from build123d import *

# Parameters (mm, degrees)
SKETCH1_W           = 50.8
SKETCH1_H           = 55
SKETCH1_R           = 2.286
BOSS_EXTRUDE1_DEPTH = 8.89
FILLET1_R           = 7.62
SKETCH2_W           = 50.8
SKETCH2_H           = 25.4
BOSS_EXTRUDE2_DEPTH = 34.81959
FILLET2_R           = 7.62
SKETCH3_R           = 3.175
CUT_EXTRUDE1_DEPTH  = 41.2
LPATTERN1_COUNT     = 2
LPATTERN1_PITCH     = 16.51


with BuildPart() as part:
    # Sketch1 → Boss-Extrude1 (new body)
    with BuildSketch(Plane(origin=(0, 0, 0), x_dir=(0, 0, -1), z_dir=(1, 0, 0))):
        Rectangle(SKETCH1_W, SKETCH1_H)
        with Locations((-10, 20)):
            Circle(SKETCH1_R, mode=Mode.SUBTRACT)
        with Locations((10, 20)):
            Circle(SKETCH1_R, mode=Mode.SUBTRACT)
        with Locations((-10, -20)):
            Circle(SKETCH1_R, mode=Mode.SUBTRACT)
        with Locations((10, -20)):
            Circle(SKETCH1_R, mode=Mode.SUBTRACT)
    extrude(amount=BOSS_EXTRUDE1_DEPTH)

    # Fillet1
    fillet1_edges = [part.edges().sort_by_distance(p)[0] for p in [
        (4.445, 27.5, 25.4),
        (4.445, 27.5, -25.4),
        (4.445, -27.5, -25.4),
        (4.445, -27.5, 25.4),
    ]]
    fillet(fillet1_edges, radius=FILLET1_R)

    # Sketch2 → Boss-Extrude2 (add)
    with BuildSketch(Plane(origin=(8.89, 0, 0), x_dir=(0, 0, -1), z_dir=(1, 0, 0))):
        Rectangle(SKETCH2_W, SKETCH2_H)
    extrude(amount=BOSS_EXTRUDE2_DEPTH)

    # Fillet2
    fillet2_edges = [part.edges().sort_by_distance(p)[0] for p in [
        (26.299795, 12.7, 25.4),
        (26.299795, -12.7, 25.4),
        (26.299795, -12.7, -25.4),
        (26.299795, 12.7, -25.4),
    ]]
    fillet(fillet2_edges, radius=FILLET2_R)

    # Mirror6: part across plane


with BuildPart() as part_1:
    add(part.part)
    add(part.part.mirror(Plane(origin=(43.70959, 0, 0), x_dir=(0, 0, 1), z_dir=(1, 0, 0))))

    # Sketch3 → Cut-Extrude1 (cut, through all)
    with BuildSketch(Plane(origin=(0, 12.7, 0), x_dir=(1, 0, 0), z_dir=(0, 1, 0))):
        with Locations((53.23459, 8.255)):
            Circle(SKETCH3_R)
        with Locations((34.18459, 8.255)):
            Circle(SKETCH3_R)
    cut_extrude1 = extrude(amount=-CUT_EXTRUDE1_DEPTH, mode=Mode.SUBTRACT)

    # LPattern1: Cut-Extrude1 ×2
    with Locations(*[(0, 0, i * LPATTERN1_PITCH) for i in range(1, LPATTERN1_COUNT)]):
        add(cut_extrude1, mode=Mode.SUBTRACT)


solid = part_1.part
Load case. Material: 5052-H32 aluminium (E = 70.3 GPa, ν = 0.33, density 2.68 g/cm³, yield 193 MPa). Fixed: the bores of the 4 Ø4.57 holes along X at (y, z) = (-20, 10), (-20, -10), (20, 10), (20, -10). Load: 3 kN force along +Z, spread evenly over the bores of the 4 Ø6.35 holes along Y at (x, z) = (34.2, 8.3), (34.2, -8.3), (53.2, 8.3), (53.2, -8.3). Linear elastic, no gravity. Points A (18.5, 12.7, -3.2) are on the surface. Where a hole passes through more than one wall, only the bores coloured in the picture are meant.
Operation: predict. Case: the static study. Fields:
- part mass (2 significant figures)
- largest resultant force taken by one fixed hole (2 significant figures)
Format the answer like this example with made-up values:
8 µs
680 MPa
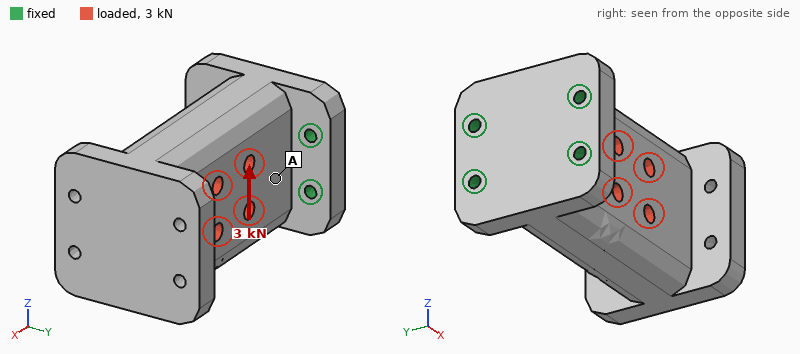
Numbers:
350 g
2.3 kN
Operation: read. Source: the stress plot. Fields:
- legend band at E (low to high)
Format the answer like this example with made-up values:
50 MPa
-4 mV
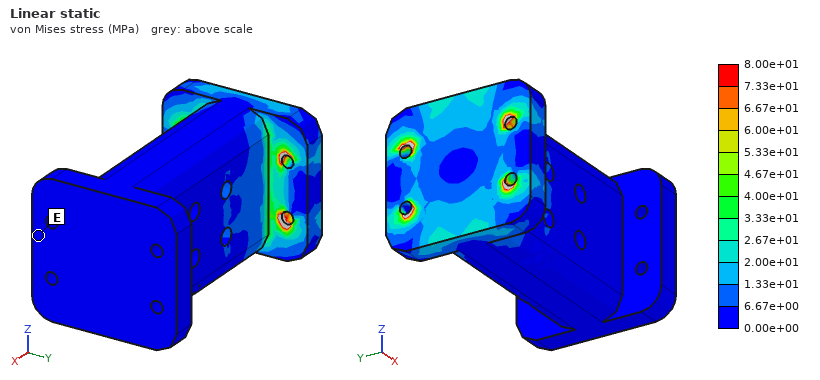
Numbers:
0.00e+00 to 6.67e+00 MPa
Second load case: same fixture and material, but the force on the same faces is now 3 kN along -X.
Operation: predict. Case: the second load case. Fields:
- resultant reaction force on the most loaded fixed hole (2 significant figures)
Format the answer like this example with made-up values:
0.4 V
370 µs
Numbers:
790 N
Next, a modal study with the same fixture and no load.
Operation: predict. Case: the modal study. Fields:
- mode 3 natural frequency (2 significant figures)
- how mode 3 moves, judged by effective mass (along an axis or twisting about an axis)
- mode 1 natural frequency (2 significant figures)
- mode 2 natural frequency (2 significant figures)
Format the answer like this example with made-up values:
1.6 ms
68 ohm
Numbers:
5500 Hz
twisting about X
1800 Hz
1900 Hz
